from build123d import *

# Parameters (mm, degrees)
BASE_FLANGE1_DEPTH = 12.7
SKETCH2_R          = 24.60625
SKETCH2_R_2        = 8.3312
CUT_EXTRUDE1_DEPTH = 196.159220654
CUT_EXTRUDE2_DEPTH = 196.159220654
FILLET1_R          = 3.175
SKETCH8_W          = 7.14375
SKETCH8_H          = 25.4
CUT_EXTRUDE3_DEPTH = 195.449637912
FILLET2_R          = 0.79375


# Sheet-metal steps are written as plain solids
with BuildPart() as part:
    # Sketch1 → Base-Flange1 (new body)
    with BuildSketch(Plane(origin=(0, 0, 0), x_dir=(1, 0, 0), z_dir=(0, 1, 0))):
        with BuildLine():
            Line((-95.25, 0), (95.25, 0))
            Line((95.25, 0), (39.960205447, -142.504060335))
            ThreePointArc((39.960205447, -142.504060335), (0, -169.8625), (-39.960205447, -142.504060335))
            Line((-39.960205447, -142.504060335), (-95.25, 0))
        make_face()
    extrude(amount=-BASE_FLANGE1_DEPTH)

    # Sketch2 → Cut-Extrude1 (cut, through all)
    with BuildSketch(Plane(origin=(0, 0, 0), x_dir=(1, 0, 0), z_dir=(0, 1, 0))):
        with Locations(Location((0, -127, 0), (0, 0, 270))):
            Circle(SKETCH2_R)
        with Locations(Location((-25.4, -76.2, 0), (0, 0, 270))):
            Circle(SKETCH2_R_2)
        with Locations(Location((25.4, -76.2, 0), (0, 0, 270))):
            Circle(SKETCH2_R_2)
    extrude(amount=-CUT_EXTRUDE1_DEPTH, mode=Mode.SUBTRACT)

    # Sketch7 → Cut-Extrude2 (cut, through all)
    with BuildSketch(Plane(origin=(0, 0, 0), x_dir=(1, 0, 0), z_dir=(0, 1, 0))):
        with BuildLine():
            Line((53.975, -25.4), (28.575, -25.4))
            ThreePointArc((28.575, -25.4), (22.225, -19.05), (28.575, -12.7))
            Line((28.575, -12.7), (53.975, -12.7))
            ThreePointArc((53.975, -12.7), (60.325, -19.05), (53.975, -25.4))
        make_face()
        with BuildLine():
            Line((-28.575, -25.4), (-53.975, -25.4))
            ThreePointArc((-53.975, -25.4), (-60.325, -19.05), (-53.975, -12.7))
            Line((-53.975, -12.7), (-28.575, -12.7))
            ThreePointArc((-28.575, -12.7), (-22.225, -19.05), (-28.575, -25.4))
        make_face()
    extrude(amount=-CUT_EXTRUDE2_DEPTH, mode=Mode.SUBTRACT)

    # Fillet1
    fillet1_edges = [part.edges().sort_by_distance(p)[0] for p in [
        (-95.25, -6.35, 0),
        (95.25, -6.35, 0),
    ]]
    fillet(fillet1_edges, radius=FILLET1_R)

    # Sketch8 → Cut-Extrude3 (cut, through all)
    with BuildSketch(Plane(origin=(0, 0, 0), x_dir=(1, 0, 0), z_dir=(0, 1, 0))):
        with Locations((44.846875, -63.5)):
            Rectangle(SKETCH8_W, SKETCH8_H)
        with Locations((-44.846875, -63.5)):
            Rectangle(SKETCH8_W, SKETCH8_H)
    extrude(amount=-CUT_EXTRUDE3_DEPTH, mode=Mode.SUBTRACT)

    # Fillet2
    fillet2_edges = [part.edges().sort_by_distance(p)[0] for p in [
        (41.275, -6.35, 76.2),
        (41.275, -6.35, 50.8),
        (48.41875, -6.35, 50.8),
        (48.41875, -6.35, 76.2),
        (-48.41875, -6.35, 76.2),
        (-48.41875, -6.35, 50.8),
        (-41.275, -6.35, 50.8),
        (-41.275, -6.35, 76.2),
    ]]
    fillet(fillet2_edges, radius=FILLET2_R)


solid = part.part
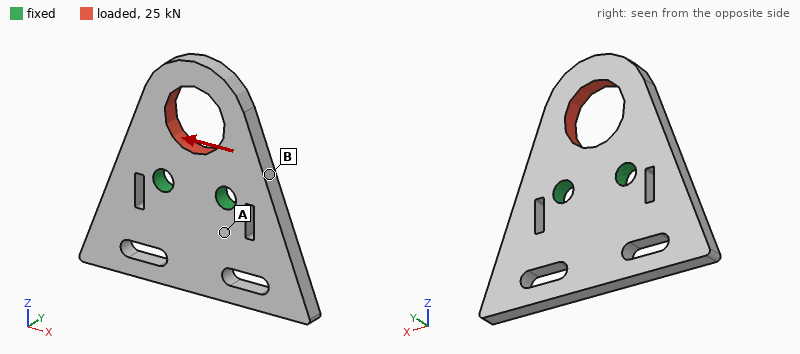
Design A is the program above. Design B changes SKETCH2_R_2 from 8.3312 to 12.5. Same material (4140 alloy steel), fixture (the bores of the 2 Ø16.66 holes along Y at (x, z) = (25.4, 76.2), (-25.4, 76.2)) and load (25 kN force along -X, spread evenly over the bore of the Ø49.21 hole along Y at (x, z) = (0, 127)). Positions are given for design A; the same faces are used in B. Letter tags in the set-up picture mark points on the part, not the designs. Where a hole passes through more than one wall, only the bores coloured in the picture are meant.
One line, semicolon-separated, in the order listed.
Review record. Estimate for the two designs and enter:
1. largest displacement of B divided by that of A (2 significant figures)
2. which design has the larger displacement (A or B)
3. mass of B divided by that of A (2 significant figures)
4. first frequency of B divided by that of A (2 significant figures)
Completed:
0.88; A; 0.97; 1.1
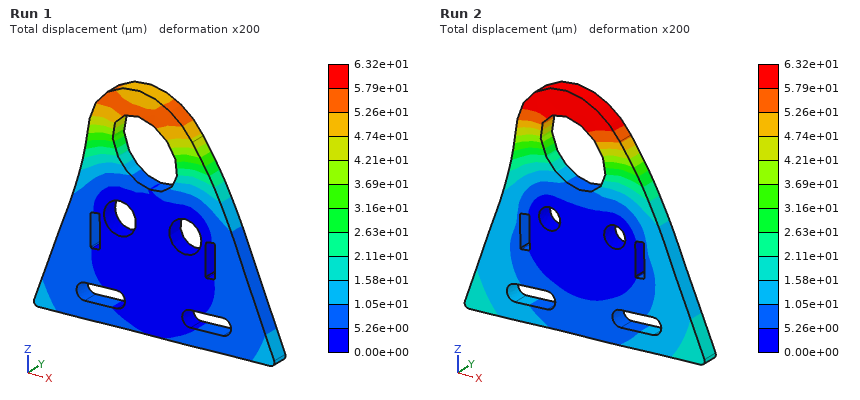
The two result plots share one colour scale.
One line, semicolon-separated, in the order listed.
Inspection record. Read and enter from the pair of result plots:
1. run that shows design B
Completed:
Run 1
